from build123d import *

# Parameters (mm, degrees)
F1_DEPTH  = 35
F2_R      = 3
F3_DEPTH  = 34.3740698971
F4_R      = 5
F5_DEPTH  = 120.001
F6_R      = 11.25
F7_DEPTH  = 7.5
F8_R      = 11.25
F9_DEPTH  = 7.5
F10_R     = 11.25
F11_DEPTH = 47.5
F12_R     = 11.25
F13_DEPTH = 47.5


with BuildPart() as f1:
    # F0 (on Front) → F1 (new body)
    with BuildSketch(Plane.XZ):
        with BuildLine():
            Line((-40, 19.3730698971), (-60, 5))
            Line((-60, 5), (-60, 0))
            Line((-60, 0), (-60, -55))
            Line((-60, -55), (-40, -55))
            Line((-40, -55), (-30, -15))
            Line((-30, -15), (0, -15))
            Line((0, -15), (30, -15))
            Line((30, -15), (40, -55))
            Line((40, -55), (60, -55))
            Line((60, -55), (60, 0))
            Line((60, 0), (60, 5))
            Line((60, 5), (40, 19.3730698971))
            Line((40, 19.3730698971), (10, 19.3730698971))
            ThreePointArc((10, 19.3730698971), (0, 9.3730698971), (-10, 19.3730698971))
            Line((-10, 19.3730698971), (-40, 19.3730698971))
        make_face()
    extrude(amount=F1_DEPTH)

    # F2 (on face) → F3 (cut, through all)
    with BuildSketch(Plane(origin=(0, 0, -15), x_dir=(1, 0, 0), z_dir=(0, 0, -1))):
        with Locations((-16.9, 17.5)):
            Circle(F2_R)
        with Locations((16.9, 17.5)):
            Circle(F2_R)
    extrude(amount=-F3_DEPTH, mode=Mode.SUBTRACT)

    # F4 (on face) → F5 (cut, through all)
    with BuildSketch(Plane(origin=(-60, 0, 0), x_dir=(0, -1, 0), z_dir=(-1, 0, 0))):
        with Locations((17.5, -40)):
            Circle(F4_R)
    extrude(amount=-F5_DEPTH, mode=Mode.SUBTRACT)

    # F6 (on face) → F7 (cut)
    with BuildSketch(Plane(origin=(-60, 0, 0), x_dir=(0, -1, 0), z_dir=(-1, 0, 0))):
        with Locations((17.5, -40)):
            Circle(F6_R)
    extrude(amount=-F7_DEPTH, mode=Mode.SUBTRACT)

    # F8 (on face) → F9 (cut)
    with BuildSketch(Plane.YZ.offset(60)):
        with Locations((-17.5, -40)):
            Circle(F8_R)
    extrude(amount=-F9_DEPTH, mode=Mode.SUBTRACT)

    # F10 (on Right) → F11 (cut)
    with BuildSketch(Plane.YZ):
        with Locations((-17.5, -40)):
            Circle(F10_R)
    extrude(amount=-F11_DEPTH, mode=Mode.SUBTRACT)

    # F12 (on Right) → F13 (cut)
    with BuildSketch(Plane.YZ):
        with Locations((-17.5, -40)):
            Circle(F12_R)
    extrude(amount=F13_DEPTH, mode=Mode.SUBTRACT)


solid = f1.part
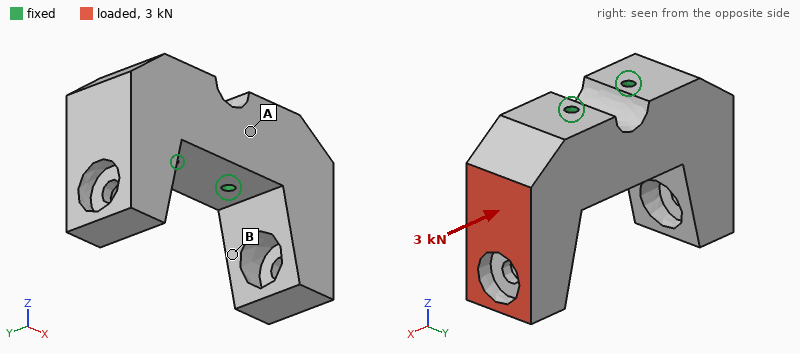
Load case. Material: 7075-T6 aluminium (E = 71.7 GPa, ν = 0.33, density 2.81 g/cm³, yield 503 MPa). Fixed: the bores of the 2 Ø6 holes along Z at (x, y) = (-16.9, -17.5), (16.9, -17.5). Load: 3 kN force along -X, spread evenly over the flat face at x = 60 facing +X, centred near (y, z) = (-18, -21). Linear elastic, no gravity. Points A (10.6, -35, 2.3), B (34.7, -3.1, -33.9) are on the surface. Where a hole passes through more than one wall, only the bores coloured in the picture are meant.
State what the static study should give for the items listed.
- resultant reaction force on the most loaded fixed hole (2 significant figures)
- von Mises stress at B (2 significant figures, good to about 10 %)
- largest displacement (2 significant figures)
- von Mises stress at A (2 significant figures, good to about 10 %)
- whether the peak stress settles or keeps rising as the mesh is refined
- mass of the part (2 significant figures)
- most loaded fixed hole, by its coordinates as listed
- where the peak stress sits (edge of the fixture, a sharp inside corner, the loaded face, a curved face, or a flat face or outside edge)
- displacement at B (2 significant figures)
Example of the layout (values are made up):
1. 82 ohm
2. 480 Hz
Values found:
1. 2.3 kN
2. 6.0 MPa
3. 27 µm
4. 2.3 MPa
5. keeps rising
6. 510 g
7. (16.9, -17.5)
8. edge of the fixture
9. 13 µm
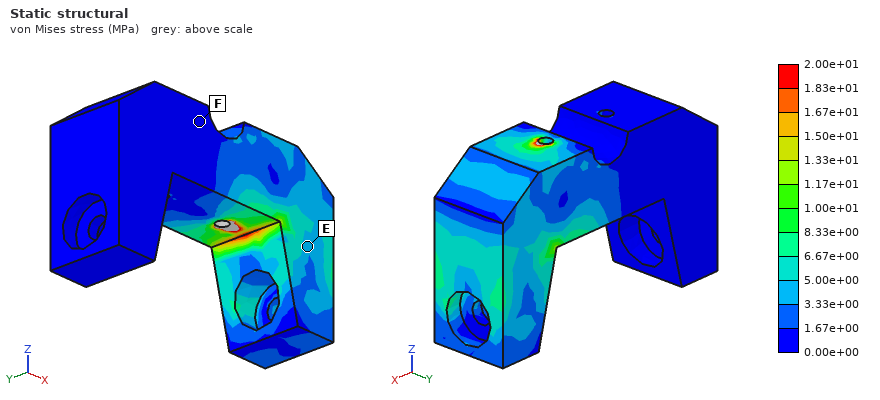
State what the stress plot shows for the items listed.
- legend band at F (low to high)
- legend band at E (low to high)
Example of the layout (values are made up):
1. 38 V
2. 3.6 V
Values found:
1. 0.00e+00 to 1.67e+00 MPa
2. 3.33e+00 to 5.00e+00 MPa
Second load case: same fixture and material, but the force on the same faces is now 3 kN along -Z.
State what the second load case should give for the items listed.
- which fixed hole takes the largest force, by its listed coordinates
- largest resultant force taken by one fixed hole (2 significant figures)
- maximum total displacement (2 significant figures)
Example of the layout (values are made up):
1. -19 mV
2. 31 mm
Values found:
1. (16.9, -17.5)
2. 3.7 kN
3. 39 µm
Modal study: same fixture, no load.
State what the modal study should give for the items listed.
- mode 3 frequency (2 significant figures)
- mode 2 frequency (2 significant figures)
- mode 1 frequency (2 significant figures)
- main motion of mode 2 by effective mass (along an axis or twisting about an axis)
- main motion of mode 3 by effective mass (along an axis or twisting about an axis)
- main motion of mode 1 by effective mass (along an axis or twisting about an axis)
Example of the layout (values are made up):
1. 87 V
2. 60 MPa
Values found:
1. 5300 Hz
2. 4700 Hz
3. 4500 Hz
4. along Y
5. along X
6. twisting about Z
